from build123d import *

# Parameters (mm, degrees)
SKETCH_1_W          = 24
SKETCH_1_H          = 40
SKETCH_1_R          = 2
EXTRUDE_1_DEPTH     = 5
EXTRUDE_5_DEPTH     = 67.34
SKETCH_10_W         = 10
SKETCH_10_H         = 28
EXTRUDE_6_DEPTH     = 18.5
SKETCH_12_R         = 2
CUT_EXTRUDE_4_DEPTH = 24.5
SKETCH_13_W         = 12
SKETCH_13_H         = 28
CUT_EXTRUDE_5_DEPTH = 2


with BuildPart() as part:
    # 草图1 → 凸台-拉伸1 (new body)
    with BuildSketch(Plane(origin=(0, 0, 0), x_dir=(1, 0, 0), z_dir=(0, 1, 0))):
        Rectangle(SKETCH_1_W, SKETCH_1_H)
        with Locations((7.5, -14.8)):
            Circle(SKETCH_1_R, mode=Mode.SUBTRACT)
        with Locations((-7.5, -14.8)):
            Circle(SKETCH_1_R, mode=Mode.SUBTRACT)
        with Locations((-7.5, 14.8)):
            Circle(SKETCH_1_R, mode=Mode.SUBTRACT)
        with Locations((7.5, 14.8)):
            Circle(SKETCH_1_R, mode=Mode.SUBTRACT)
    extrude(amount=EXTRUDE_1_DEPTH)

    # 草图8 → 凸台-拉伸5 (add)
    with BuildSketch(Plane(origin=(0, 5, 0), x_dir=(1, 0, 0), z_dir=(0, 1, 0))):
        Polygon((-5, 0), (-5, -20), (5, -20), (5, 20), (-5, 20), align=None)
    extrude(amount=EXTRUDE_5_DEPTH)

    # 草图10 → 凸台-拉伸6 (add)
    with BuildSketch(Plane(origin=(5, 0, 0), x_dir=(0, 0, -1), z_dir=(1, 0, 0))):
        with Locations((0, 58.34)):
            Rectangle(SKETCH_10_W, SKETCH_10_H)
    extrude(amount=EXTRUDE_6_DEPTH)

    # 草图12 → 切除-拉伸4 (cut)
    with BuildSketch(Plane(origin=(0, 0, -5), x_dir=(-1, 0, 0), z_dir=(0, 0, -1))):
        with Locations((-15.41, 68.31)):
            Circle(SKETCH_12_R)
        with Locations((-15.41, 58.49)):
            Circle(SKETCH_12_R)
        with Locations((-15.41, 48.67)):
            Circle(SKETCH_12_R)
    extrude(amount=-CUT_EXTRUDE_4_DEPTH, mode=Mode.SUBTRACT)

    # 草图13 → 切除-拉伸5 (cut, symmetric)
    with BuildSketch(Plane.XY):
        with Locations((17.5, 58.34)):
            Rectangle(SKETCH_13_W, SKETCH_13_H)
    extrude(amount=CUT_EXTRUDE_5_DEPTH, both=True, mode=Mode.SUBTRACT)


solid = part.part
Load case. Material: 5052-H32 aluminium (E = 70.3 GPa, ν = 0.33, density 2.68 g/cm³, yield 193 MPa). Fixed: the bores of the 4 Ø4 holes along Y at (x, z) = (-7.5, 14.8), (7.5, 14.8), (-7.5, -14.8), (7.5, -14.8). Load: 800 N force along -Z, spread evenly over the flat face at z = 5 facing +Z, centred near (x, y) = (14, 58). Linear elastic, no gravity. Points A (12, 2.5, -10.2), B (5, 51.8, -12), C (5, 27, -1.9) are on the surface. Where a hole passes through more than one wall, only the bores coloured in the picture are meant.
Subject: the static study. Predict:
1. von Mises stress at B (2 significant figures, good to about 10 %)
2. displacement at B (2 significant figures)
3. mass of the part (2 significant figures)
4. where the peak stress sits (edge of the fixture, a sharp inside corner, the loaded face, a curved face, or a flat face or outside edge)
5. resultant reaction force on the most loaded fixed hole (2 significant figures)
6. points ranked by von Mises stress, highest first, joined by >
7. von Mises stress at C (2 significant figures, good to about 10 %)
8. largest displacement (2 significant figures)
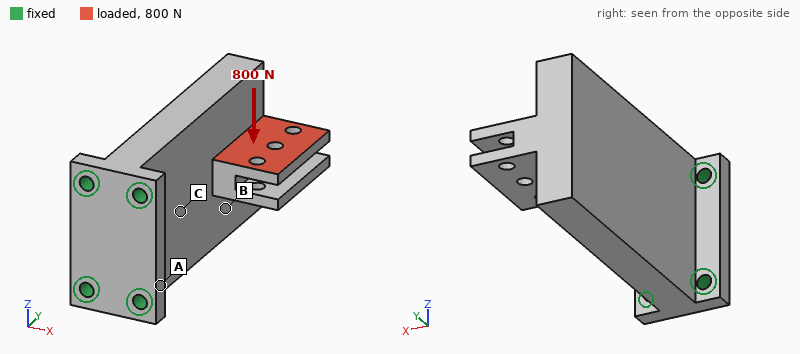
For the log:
13 MPa
0.032 mm
94 g
edge of the fixture
1.1 kN
C > B > A
20 MPa
0.13 mm
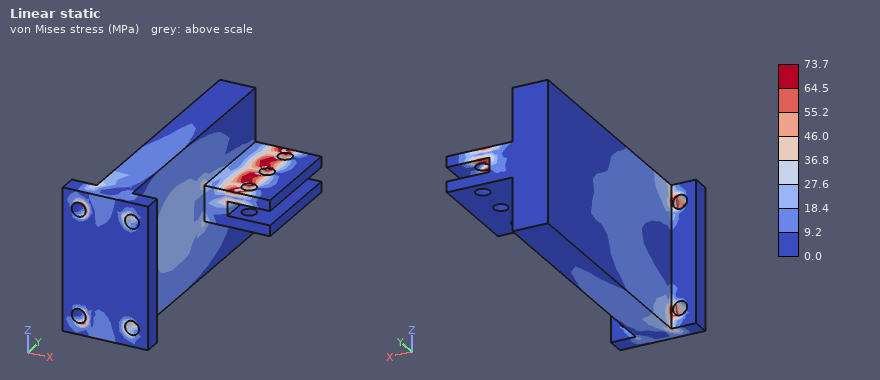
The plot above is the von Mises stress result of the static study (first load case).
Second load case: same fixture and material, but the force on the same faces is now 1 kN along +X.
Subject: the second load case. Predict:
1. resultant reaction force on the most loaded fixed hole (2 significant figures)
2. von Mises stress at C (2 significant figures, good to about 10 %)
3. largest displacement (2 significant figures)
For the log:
2.3 kN
46 MPa
0.44 mm
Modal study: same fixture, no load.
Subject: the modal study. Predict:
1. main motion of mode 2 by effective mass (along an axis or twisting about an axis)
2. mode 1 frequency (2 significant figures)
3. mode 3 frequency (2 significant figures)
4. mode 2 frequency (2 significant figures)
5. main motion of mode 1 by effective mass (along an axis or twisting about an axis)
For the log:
along Z
1400 Hz
5200 Hz
4000 Hz
along X
